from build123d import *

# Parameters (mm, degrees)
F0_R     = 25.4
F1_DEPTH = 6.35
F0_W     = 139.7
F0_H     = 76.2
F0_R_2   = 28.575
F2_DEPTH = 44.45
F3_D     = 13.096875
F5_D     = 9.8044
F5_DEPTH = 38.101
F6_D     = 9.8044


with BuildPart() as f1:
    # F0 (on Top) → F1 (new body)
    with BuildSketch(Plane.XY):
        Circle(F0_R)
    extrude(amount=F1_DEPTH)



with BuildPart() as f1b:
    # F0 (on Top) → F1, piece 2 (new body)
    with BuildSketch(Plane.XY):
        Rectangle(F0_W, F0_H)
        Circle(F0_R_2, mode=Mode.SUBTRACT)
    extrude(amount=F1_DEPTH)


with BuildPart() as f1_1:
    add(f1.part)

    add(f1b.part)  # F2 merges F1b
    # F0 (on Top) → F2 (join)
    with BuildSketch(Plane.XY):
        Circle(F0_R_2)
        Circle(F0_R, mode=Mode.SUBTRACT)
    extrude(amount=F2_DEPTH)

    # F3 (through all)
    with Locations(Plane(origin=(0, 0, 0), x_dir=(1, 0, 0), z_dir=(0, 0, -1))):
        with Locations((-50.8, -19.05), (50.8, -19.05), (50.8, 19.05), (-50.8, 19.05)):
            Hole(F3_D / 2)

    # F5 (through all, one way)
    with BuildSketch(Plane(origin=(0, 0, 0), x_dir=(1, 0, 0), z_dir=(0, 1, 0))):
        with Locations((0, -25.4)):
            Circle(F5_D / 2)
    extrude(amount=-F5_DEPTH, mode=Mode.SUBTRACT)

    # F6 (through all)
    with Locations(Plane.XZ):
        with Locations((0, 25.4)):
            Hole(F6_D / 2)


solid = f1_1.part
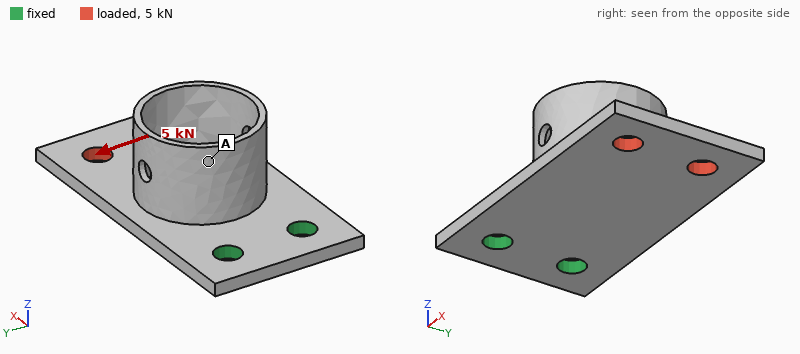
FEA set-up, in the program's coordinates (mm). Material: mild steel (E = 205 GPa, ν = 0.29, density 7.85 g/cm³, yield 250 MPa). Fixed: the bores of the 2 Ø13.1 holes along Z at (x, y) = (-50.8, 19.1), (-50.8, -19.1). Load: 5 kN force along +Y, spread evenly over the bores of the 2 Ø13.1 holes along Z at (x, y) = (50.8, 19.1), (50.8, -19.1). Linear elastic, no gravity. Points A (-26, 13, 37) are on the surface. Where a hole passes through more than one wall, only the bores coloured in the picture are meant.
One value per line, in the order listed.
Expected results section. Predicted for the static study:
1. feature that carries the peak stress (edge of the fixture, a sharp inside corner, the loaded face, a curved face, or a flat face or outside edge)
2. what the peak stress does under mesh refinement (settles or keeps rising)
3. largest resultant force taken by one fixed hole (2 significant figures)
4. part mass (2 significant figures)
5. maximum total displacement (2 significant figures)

edge of the fixture
keeps rising
11 kN
660 g
73 µm
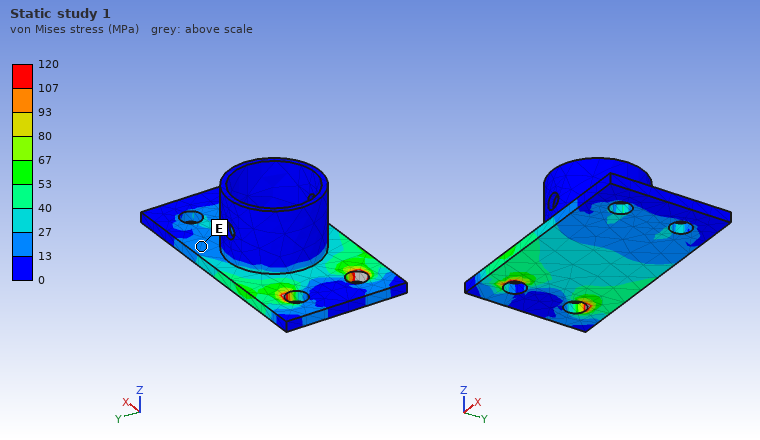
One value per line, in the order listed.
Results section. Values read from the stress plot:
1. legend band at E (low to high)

13 to 27 MPa
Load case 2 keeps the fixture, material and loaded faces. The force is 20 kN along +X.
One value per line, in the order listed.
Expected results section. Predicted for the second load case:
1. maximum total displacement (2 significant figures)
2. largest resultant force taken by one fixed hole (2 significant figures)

37 µm
10 kN
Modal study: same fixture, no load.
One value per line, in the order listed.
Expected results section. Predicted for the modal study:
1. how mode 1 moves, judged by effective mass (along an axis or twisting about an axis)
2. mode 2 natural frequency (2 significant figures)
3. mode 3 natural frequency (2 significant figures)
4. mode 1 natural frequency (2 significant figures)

along Z
1500 Hz
2500 Hz
410 Hz
